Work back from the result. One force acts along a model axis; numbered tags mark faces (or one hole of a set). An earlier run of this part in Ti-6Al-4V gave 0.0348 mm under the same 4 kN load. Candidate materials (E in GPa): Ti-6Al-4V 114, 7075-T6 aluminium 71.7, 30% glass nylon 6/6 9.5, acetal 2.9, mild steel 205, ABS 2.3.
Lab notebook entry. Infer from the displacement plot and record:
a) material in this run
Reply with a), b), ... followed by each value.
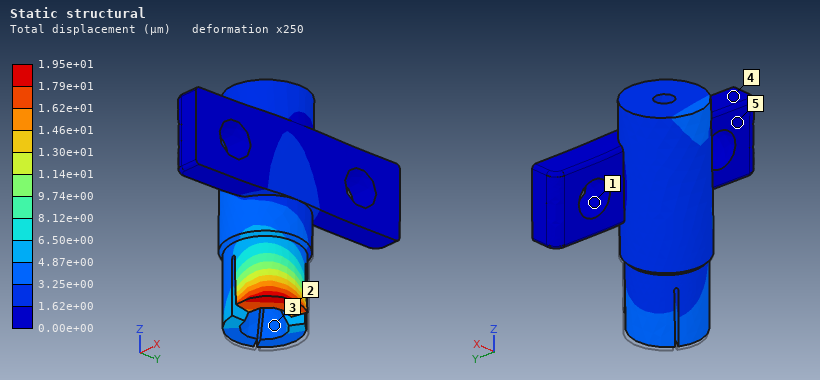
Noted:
a) mild steel
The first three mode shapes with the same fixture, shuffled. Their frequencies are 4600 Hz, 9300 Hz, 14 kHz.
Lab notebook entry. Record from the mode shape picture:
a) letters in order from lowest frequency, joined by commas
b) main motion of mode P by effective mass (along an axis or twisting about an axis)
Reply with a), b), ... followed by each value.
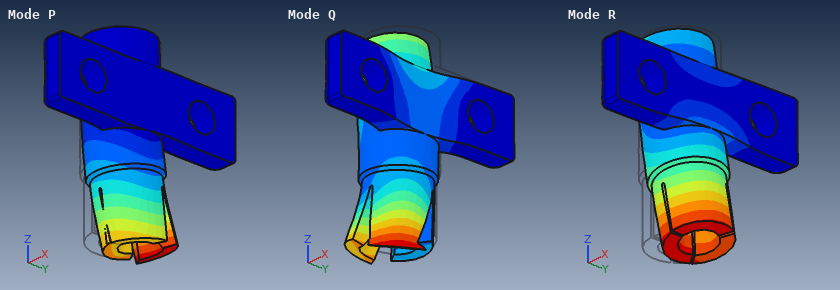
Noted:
a) R, P, Q
b) along Y
